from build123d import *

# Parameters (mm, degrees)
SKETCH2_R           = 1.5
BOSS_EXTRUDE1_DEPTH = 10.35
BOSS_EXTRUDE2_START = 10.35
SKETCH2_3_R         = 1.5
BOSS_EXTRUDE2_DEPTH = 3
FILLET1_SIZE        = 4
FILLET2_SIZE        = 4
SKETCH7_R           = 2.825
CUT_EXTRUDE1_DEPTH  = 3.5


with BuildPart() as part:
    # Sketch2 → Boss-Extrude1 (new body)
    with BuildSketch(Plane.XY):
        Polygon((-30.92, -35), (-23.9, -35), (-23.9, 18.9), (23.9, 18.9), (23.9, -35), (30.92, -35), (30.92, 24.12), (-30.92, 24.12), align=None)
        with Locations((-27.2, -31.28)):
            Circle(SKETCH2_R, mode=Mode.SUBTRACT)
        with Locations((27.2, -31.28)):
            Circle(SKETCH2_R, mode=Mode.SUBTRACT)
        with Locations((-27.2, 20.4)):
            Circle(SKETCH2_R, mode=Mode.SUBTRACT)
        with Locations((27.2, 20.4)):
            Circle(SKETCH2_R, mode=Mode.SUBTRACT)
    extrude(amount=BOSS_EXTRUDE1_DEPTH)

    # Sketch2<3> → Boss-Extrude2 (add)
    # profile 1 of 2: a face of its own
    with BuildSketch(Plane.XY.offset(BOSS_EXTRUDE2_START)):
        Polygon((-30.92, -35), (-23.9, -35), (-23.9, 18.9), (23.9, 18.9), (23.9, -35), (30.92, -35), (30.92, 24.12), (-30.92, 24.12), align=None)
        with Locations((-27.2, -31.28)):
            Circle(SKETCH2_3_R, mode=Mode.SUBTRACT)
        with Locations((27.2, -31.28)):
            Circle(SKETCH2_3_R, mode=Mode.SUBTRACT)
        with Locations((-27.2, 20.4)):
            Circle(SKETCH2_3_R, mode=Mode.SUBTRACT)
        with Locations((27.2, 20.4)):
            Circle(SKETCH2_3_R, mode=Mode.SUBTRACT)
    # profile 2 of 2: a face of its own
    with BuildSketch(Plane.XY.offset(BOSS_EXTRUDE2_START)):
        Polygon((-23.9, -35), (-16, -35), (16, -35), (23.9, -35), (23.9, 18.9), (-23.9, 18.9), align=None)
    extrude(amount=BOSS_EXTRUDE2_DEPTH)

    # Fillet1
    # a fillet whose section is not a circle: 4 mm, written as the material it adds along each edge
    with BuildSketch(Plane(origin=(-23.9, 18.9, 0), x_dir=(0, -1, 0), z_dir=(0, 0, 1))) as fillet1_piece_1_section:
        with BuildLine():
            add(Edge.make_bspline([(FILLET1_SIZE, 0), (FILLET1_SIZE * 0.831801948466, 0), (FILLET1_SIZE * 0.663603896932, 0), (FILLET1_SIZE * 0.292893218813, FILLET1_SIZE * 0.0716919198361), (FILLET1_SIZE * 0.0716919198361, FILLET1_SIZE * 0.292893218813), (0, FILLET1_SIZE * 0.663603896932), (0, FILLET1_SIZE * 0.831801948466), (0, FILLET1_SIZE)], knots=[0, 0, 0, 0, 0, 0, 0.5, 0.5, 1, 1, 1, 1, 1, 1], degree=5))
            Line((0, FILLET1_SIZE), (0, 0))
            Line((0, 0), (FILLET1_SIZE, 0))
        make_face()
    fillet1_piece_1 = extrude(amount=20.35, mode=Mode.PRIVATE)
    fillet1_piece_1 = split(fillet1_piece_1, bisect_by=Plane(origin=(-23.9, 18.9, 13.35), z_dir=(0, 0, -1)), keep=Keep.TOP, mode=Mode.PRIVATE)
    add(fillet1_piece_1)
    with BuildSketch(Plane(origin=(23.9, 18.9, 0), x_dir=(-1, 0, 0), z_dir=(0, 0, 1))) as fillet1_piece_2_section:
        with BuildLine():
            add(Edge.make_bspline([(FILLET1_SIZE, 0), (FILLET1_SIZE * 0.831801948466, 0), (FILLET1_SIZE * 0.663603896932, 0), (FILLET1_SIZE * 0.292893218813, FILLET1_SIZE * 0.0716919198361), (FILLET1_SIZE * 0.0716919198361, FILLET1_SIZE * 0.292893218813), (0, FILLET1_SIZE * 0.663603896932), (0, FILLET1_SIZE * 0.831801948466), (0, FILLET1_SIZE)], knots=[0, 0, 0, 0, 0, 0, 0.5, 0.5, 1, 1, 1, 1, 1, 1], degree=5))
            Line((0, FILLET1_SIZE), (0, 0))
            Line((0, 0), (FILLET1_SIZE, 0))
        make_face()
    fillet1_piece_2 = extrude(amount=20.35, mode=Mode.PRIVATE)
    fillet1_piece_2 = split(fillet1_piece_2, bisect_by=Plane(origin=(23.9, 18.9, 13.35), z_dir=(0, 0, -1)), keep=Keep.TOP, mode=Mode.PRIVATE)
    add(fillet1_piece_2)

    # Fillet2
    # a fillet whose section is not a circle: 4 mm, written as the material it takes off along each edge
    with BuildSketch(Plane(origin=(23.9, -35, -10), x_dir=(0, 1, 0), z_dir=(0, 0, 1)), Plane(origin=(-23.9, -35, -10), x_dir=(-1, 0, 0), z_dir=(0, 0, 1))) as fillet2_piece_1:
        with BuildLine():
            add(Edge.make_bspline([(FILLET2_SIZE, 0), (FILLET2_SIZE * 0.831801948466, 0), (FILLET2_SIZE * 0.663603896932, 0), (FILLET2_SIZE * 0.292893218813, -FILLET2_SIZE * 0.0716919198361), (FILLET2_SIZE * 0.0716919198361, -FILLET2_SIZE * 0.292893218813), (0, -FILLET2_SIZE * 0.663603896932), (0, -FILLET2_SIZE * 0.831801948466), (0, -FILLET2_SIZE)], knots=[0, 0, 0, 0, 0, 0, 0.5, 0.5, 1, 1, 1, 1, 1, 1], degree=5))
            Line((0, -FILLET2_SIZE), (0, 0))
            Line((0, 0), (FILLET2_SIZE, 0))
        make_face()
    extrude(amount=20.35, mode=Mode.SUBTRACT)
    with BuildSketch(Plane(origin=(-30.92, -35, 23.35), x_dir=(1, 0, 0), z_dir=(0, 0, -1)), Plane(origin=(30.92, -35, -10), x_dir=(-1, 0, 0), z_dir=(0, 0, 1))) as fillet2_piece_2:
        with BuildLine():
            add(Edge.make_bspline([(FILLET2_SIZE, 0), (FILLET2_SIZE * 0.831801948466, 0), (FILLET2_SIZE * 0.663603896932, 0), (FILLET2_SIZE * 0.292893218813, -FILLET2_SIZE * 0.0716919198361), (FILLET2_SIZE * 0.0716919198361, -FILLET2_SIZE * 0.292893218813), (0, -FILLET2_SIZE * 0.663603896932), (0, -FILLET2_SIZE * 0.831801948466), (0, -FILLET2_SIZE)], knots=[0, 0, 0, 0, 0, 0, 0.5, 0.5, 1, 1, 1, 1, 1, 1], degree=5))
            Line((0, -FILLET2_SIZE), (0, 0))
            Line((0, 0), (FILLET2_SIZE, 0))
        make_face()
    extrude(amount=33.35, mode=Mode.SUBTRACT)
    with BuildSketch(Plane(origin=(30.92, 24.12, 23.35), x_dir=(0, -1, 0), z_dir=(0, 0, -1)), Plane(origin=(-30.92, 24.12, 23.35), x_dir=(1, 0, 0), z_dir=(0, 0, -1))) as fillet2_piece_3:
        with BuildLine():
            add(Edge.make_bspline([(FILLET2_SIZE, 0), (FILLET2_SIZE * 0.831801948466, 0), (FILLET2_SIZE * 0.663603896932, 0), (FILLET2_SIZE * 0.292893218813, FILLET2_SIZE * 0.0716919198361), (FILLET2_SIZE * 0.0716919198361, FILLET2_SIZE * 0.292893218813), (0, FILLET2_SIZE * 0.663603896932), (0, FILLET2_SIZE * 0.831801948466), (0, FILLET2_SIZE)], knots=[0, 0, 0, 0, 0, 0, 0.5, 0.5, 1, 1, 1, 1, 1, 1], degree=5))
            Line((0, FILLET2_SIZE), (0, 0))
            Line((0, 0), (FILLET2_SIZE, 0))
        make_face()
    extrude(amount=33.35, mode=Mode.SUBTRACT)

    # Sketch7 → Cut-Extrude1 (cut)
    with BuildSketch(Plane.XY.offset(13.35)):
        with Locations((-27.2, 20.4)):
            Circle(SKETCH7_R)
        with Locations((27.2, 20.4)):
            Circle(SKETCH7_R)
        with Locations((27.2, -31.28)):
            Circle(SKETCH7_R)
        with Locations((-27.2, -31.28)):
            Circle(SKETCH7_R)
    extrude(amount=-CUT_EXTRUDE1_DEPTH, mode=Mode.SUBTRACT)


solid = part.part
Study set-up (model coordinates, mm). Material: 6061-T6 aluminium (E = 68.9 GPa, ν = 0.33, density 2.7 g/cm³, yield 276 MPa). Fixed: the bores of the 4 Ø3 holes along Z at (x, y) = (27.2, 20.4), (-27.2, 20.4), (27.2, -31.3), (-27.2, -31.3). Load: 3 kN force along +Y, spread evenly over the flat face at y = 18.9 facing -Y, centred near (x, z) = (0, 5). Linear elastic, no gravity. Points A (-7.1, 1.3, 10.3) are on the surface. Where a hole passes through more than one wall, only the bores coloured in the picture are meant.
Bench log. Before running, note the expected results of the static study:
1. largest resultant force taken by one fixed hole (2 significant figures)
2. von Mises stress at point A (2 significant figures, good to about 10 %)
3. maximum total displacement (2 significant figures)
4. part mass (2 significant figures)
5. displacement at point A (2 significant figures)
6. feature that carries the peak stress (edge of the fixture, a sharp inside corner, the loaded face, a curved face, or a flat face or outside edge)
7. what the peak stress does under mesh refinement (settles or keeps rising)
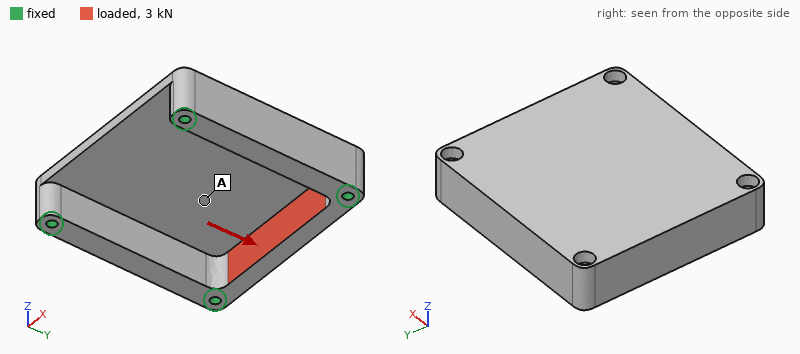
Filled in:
1.1 kN
16 MPa
76 µm
58 g
19 µm
edge of the fixture
keeps rising
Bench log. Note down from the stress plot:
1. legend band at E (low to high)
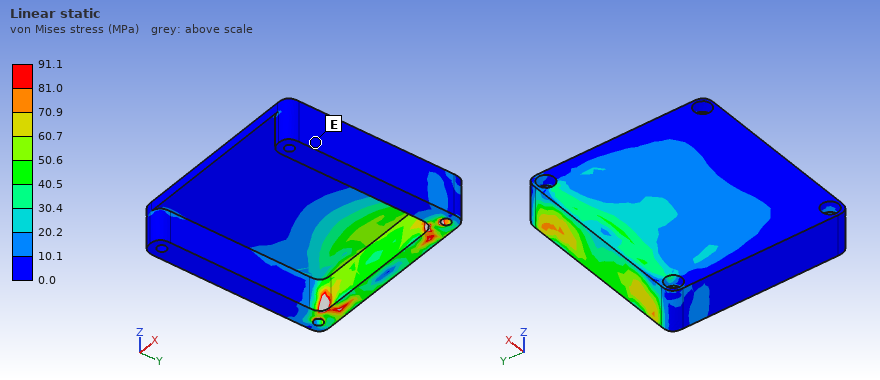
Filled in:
0.0 to 10.1 MPa
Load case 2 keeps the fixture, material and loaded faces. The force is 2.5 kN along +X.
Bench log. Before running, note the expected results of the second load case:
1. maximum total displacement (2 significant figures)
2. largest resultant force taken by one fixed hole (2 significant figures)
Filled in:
5.8 µm
1.2 kN
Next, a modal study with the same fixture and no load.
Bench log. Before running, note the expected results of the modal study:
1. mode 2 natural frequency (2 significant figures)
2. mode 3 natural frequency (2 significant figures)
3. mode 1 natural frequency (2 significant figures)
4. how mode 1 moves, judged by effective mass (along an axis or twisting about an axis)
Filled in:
8700 Hz
13 kHz
5800 Hz
along Z
